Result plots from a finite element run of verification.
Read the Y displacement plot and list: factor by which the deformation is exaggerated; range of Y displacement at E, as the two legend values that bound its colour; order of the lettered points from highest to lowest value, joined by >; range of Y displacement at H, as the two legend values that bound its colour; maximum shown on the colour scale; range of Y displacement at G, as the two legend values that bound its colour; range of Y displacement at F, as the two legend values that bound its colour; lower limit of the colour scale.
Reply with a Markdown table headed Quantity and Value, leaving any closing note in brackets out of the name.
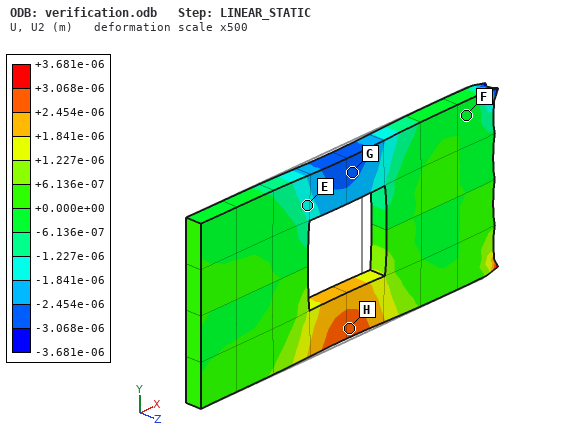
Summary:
| Quantity | Value |
|---|---|
| factor by which the deformation is exaggerated | 500 |
| range of Y displacement at E, as the two legend values that bound its colour | -1.841e-06 to -1.227e-06 m |
| order of the lettered points from highest to lowest value, joined by > | H > F > E > G |
| range of Y displacement at H, as the two legend values that bound its colour | +2.454e-06 to +3.068e-06 m |
| maximum shown on the colour scale | +3.681e-06 m |
| range of Y displacement at G, as the two legend values that bound its colour | -3.068e-06 to -2.454e-06 m |
| range of Y displacement at F, as the two legend values that bound its colour | -6.136e-07 to +0.000e+00 m |
| lower limit of the colour scale | -3.681e-06 m |
